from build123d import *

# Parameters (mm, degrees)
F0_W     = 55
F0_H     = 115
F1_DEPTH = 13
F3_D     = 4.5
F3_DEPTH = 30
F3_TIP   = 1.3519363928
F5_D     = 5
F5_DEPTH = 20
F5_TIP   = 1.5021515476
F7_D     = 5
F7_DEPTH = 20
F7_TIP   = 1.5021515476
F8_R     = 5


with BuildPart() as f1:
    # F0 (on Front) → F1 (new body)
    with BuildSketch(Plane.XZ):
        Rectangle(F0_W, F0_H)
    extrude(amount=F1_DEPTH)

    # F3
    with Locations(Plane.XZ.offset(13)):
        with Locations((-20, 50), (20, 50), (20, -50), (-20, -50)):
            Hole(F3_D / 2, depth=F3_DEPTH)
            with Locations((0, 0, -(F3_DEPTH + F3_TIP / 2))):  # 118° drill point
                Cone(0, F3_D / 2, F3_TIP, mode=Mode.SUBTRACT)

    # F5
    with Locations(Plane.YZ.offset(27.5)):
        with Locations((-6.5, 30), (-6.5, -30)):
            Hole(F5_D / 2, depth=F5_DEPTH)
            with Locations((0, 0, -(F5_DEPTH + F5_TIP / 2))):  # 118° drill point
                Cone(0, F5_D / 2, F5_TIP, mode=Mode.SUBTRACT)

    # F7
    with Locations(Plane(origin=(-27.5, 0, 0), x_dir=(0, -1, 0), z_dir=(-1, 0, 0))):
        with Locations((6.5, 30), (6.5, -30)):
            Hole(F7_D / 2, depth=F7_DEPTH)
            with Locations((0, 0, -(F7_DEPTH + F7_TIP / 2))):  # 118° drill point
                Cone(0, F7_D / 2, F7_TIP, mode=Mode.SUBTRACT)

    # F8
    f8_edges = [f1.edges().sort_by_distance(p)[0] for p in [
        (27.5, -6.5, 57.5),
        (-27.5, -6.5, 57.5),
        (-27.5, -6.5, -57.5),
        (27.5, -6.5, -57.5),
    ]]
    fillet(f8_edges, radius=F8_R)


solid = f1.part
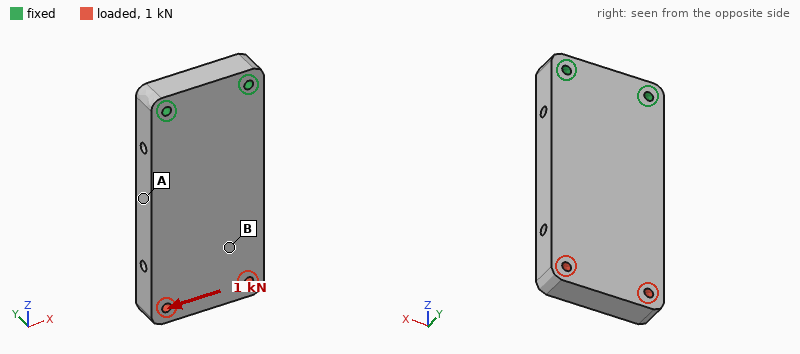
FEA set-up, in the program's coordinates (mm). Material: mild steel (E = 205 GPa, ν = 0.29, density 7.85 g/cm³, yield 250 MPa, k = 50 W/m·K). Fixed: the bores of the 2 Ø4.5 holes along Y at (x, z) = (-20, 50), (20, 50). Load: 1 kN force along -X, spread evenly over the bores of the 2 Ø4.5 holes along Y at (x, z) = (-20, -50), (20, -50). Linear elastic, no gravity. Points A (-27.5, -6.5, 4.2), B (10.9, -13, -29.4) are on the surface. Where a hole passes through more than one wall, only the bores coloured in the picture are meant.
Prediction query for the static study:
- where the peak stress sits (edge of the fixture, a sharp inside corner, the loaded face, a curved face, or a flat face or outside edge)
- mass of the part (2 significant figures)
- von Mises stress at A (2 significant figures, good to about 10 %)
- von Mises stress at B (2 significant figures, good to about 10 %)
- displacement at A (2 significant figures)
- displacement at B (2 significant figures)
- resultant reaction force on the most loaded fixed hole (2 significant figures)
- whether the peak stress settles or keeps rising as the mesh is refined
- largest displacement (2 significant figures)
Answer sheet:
edge of the fixture
620 g
8.3 MPa
3.9 MPa
5.2 µm
9.2 µm
2.5 kN
keeps rising
14 µm
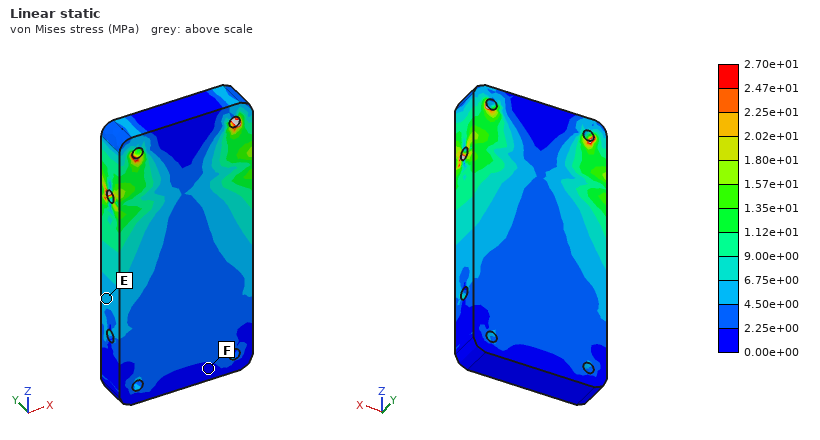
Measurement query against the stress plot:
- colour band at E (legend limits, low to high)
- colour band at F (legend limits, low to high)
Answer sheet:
4.50e+00 to 6.75e+00 MPa
0.00e+00 to 2.25e+00 MPa
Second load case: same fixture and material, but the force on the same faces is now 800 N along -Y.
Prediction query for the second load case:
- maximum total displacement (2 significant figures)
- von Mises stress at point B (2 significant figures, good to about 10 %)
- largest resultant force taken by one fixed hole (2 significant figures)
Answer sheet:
0.17 mm
11 MPa
400 N
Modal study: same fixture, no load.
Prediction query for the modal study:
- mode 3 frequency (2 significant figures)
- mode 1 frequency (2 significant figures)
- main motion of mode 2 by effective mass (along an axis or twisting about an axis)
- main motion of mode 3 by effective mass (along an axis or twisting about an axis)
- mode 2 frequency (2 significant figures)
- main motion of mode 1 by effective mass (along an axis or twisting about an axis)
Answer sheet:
3500 Hz
860 Hz
along X
twisting about Z
3200 Hz
along Y
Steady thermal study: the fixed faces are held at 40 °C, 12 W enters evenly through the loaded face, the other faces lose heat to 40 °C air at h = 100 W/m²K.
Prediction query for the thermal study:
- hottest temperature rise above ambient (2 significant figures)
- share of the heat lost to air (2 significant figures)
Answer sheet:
16 K
82 %
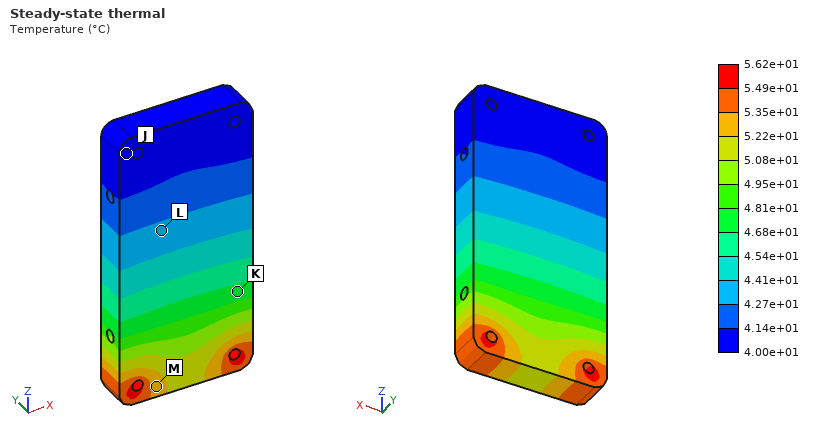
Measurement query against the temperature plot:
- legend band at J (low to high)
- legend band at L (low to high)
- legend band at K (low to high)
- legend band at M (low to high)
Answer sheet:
4.00e+01 to 4.14e+01 °C
4.27e+01 to 4.41e+01 °C
4.68e+01 to 4.81e+01 °C
5.22e+01 to 5.35e+01 °C
